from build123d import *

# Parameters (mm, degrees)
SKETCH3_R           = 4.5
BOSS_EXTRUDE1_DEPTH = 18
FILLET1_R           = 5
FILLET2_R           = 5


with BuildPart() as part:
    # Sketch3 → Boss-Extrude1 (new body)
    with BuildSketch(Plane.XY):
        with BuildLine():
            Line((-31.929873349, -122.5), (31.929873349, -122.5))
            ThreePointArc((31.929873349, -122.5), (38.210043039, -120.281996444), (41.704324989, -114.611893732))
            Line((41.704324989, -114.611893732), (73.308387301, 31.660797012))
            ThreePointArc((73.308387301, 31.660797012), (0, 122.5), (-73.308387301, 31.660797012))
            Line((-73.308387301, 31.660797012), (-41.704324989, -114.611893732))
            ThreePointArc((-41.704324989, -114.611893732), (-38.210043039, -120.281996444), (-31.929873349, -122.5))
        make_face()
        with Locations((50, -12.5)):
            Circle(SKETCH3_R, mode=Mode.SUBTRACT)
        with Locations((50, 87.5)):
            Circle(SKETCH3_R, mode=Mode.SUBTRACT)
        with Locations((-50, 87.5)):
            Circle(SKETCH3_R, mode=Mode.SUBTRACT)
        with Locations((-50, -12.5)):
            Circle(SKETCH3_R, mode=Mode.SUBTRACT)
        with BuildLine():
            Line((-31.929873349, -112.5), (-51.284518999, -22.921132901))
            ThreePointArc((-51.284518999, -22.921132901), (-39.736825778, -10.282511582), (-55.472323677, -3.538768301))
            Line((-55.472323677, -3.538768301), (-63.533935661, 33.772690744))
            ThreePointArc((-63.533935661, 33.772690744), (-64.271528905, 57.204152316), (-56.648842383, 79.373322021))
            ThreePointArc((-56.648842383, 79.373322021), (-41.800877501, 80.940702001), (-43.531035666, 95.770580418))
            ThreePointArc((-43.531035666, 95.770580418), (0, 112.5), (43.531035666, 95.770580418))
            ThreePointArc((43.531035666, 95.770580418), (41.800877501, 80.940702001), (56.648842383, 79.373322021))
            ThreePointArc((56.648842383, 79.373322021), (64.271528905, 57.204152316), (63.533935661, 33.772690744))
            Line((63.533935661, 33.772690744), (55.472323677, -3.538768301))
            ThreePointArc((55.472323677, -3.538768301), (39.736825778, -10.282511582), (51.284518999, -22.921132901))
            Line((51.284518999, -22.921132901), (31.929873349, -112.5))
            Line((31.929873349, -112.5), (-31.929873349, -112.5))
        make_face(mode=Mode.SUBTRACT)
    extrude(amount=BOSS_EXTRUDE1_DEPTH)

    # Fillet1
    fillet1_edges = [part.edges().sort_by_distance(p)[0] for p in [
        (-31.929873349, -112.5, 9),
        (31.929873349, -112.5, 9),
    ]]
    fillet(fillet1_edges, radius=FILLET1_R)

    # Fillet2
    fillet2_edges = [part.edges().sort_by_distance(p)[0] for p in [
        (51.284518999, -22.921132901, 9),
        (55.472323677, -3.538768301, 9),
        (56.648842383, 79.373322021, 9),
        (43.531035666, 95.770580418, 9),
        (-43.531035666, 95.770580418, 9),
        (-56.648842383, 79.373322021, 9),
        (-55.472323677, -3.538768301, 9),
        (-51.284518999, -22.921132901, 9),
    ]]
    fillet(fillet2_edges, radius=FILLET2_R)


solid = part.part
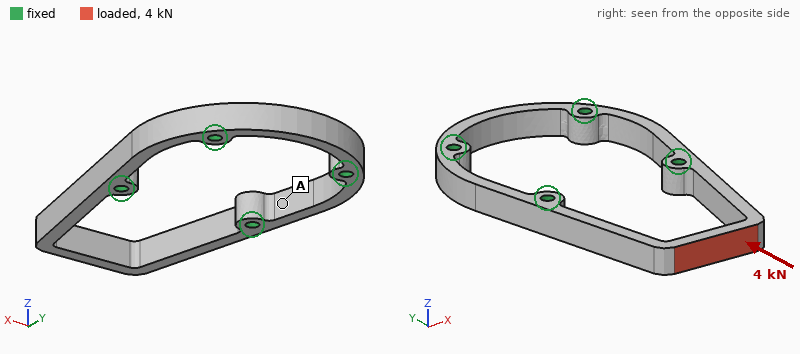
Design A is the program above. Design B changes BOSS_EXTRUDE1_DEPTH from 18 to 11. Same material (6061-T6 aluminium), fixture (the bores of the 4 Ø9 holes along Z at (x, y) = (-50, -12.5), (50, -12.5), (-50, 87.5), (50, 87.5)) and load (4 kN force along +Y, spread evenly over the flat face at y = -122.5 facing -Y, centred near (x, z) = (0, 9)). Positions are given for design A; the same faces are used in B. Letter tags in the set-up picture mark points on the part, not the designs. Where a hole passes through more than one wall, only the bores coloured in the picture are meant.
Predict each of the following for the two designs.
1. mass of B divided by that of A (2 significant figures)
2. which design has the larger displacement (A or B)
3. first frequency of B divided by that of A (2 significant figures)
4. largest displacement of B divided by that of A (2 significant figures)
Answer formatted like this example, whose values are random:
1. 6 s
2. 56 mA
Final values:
1. 0.61
2. B
3. 0.63
4. 1.6
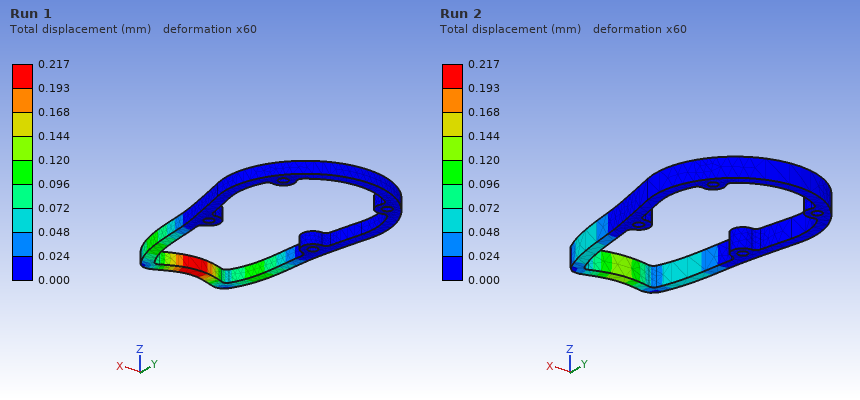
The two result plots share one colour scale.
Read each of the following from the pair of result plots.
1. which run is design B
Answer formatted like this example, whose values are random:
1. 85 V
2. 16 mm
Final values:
1. Run 1
